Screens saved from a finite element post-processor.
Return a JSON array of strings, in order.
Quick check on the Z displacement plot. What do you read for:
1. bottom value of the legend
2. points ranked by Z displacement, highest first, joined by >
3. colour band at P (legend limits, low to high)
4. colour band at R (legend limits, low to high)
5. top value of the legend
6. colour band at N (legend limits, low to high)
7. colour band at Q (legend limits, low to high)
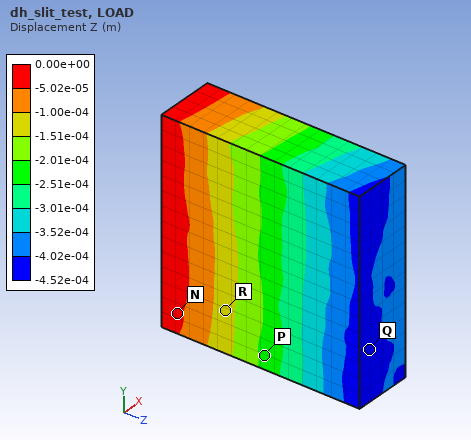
["-4.52e-04 m", "N > R > P > Q", "-2.51e-04 to -2.01e-04 m", "-1.51e-04 to -1.00e-04 m", "0.00e+00 m", "-5.02e-05 to 0.00e+00 m", "-4.52e-04 to -4.02e-04 m"]
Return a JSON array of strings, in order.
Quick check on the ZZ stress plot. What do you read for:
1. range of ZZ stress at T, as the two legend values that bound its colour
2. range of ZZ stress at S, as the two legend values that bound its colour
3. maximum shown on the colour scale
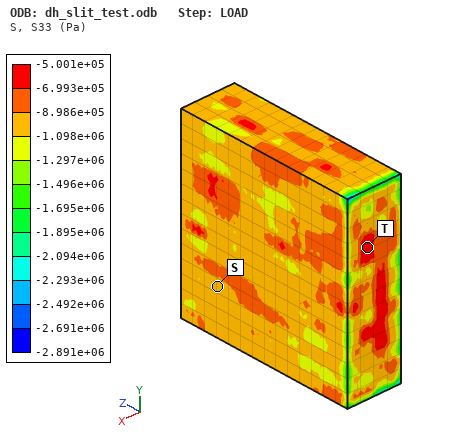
["-6.993e+05 to -5.001e+05 Pa", "-1.098e+06 to -8.986e+05 Pa", "-5.001e+05 Pa"]
